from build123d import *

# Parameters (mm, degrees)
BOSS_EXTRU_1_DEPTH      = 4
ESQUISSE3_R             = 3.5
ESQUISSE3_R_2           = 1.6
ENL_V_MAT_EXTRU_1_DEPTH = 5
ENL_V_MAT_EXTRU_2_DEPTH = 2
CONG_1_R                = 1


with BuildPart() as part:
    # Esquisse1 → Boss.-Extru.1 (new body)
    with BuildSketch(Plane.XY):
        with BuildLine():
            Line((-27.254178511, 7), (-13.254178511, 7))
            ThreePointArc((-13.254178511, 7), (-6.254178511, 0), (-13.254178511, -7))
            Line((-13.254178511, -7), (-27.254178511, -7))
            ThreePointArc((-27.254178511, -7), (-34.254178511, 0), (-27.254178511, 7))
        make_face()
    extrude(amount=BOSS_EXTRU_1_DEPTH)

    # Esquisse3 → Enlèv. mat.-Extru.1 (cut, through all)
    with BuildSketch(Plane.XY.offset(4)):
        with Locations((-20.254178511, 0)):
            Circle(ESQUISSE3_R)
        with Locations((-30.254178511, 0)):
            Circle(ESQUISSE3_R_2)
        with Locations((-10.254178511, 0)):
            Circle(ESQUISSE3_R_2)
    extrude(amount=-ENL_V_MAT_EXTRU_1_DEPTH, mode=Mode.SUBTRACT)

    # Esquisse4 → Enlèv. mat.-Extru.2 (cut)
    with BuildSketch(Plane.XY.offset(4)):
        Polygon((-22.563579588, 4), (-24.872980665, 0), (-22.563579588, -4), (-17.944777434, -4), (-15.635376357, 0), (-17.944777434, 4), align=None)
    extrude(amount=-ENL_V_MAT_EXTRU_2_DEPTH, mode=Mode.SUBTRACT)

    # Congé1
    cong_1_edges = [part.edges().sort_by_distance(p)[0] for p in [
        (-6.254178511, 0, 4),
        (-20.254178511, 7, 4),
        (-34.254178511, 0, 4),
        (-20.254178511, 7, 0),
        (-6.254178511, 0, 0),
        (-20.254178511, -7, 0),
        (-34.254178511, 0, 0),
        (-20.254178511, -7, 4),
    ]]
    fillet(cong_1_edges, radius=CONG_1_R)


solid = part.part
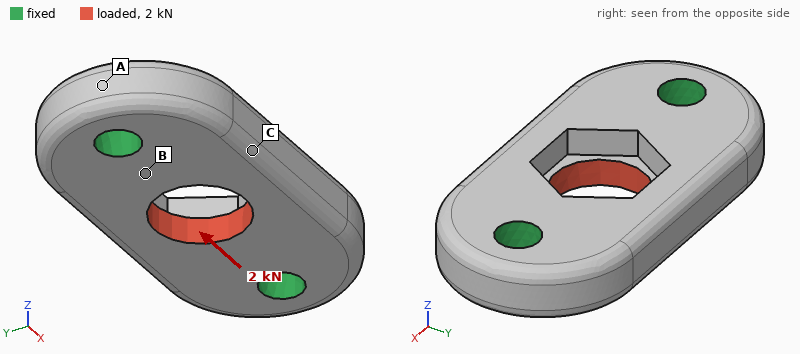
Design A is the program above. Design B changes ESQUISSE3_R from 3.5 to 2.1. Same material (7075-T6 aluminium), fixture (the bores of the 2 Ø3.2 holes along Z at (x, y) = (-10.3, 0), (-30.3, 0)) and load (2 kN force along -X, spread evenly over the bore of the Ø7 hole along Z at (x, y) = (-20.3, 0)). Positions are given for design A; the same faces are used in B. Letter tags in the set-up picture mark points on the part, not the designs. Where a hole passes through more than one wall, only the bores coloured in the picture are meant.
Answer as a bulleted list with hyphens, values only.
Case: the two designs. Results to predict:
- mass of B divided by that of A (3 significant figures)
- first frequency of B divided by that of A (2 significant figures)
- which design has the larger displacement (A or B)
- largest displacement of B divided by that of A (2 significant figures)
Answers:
- 1.04
- 1.00
- B
- 1.3
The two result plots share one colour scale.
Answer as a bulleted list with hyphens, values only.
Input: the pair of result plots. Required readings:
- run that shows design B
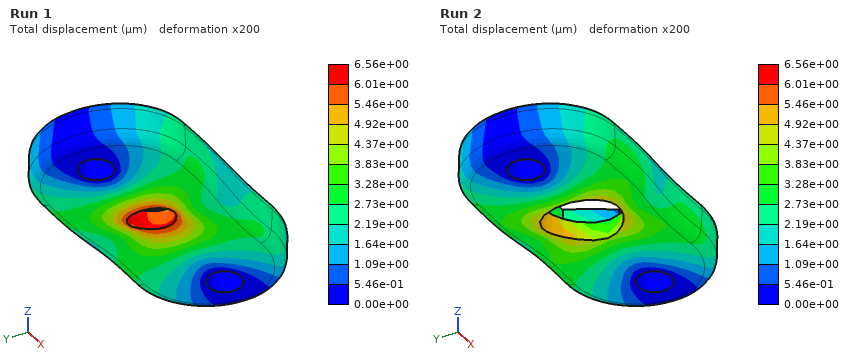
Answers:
- Run 1
